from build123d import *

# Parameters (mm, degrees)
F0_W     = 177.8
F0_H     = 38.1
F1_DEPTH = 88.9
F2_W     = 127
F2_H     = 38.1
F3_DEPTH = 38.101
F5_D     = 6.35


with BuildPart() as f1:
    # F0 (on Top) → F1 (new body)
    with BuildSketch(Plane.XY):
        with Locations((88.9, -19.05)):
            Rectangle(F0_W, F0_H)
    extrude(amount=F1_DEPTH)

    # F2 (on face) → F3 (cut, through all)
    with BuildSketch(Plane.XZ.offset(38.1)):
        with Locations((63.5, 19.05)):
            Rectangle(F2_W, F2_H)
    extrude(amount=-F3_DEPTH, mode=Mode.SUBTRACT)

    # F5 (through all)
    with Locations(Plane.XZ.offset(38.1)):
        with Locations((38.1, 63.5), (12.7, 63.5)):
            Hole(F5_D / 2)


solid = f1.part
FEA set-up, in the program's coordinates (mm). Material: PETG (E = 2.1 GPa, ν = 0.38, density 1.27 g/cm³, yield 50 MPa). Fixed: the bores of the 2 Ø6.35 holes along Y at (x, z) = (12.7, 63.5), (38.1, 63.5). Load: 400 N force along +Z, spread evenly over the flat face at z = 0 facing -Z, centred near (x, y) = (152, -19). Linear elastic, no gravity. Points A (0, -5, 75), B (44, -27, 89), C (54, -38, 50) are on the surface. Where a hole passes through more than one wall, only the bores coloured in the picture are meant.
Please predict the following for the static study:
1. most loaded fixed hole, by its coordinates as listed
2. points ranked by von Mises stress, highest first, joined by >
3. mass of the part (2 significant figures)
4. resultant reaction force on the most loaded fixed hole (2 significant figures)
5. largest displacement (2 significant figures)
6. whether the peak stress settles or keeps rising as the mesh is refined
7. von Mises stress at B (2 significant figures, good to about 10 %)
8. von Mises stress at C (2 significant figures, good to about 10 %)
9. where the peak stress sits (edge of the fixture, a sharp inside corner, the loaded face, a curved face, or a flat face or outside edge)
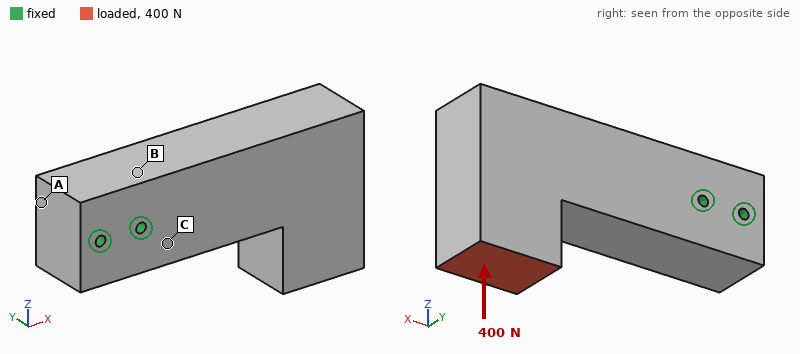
(38.1, 63.5)
B > C > A
530 g
1.8 kN
0.68 mm
keeps rising
2.9 MPa
1.2 MPa
edge of the fixture
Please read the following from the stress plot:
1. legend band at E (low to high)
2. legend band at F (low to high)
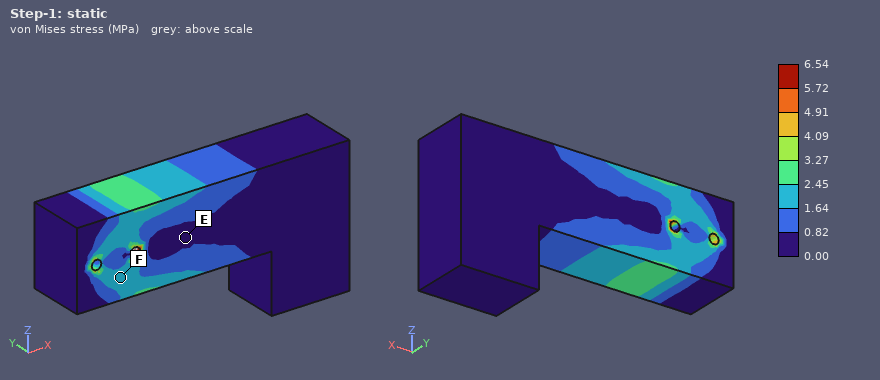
0.00 to 0.82 MPa
1.64 to 2.45 MPa
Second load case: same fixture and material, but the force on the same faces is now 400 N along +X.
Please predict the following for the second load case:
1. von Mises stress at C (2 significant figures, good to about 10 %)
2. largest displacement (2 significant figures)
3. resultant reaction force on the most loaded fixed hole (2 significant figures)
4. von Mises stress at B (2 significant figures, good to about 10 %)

0.94 MPa
0.52 mm
850 N
1.5 MPa
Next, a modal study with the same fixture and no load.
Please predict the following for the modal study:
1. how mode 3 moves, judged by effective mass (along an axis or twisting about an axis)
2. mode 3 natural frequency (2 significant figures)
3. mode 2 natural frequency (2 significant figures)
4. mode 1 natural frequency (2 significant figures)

twisting about X
680 Hz
280 Hz
270 Hz
